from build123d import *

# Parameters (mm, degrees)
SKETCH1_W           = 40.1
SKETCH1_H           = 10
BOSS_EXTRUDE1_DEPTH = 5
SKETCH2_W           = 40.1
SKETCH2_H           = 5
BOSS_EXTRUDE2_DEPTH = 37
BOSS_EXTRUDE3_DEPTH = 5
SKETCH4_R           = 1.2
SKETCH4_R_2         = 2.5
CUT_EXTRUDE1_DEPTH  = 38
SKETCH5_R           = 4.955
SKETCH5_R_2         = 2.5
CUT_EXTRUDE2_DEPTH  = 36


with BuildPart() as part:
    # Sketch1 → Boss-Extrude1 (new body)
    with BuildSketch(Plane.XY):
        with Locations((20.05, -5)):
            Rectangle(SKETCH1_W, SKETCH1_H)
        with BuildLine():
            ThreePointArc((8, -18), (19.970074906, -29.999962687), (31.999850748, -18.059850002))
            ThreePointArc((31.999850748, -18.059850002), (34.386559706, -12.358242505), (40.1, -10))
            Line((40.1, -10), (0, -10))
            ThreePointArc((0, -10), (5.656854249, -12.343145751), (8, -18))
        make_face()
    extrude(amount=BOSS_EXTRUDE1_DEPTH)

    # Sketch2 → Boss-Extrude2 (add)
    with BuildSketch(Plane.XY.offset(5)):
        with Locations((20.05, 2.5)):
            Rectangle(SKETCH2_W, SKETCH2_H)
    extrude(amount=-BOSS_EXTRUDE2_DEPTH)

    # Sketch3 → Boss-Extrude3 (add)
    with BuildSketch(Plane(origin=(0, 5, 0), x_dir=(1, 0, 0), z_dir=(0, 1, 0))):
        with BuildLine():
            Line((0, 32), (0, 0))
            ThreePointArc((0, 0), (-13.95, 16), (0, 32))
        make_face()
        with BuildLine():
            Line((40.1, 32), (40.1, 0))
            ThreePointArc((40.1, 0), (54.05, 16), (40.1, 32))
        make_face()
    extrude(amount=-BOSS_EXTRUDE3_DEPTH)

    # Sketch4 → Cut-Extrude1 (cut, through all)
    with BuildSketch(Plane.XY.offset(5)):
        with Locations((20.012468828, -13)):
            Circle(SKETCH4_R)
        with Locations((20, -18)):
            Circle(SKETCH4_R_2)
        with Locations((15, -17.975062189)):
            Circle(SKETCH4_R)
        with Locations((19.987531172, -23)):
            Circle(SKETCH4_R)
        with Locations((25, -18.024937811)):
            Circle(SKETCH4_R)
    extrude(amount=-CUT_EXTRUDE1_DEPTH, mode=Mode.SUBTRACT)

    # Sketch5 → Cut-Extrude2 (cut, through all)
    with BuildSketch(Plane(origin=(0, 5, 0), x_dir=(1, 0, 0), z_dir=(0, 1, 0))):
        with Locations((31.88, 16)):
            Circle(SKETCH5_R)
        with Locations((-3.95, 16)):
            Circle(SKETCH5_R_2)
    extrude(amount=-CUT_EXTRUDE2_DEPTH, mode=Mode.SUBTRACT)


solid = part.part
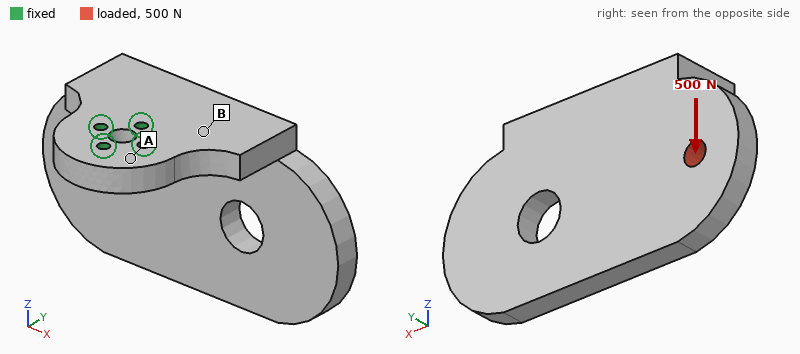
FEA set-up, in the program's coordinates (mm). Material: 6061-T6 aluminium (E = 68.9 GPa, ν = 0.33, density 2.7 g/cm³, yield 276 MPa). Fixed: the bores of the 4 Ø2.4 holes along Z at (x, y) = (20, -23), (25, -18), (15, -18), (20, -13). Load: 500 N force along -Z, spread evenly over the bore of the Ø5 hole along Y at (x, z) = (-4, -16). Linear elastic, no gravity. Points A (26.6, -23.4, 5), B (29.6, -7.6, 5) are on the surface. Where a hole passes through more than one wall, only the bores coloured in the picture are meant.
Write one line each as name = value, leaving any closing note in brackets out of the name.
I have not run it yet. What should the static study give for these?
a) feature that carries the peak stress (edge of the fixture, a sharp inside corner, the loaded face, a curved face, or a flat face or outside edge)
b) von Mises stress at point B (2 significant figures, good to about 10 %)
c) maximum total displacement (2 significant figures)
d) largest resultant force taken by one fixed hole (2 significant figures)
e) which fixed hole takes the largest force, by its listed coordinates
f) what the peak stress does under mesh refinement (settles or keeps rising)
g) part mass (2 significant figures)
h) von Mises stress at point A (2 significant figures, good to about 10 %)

feature that carries the peak stress = edge of the fixture
von Mises stress at point B = 52 MPa
maximum total displacement = 0.28 mm
largest resultant force taken by one fixed hole = 770 N
which fixed hole takes the largest force, by its listed coordinates = (20, -13)
what the peak stress does under mesh refinement = keeps rising
part mass = 39 g
von Mises stress at point A = 17 MPa
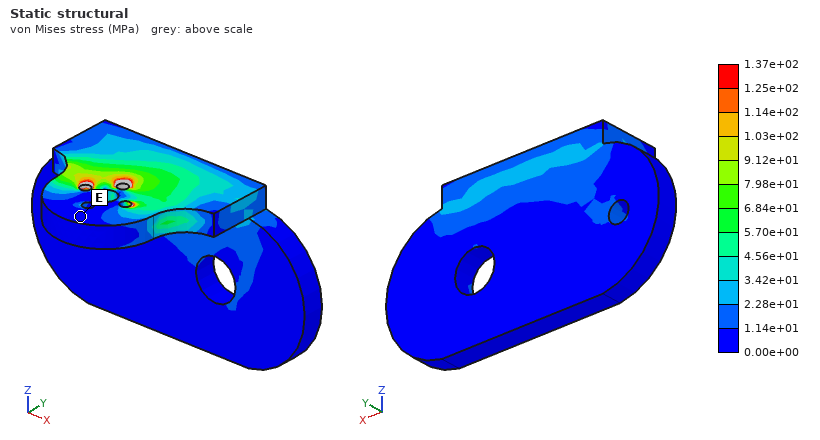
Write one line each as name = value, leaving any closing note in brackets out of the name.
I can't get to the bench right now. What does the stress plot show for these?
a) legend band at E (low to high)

legend band at E = 0.00e+00 to 1.14e+01 MPa
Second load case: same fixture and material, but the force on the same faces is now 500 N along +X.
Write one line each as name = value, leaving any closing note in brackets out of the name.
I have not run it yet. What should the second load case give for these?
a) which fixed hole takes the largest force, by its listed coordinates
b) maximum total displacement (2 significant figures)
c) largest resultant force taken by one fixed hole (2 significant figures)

which fixed hole takes the largest force, by its listed coordinates = (20, -13)
maximum total displacement = 0.16 mm
largest resultant force taken by one fixed hole = 690 N
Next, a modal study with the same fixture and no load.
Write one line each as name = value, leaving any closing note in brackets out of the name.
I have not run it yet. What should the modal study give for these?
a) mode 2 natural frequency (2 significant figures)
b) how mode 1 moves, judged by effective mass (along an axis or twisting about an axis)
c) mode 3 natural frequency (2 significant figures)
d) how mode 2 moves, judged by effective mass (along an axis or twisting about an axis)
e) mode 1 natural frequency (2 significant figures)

mode 2 natural frequency = 1800 Hz
how mode 1 moves, judged by effective mass = along Y
mode 3 natural frequency = 3500 Hz
how mode 2 moves, judged by effective mass = along X
mode 1 natural frequency = 1500 Hz
